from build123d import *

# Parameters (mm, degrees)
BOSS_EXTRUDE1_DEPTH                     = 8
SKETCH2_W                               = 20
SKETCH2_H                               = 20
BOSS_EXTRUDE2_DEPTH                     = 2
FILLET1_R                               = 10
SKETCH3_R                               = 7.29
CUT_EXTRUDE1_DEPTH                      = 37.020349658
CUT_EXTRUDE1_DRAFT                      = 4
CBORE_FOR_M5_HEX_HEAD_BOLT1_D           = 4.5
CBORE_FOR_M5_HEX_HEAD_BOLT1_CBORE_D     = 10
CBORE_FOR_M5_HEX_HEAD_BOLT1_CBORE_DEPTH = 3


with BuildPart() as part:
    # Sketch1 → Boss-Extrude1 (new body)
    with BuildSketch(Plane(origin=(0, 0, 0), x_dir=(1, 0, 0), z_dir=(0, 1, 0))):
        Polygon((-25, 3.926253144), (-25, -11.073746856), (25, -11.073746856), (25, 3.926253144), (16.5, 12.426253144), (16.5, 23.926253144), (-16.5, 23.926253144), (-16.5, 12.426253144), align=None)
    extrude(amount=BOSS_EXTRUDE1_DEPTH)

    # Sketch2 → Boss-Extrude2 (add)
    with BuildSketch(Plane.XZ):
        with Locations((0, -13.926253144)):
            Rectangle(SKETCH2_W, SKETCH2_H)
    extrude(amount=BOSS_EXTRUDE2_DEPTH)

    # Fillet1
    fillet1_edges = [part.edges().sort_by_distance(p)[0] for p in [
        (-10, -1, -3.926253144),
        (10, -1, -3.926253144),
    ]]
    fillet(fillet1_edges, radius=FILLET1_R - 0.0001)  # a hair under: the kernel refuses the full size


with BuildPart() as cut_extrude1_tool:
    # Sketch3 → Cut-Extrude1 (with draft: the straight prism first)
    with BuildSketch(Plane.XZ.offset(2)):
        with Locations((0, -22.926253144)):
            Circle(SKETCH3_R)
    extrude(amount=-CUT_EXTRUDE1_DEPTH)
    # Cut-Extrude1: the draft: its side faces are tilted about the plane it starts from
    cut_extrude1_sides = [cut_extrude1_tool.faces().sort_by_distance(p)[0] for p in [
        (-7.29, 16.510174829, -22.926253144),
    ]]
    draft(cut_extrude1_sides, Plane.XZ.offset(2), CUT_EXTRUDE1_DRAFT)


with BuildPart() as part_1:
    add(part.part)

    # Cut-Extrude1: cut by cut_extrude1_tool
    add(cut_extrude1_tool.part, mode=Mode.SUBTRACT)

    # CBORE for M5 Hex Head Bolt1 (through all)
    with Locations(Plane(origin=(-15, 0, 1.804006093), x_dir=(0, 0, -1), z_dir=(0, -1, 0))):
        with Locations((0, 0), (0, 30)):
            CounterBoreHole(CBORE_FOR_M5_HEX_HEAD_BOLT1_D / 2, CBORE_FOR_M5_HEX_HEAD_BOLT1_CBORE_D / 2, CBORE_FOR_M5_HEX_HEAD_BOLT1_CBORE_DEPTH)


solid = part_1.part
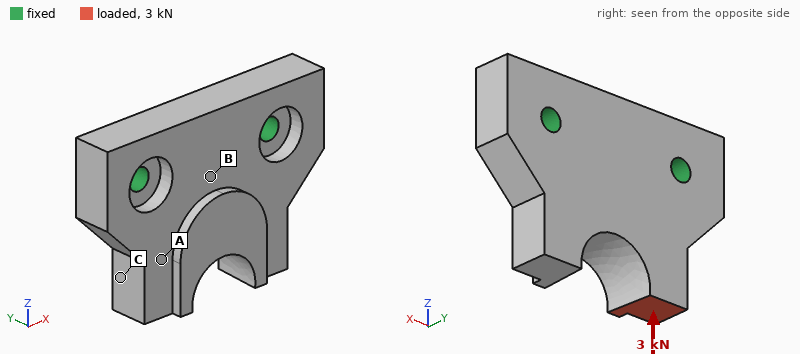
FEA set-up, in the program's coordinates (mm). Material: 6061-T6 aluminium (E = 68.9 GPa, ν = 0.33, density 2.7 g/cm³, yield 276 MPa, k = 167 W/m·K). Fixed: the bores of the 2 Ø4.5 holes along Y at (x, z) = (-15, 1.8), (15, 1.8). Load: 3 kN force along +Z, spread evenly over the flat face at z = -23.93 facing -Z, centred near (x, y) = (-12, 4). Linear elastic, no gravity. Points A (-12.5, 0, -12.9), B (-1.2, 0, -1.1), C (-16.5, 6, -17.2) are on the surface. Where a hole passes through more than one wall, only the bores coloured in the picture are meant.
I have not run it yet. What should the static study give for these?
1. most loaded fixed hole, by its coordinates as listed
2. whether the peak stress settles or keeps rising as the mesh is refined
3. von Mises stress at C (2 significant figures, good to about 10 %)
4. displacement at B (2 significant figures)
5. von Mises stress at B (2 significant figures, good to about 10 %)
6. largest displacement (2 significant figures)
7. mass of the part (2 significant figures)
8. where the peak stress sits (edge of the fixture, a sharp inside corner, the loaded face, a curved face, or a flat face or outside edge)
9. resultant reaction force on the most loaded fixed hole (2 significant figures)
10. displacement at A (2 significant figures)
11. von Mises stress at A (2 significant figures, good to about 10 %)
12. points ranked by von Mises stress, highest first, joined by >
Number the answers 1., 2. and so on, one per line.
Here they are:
1. (-15, 1.8)
2. keeps rising
3. 48 MPa
4. 6.3 µm
5. 10 MPa
6. 30 µm
7. 29 g
8. edge of the fixture
9. 2.6 kN
10. 16 µm
11. 29 MPa
12. C > A > B
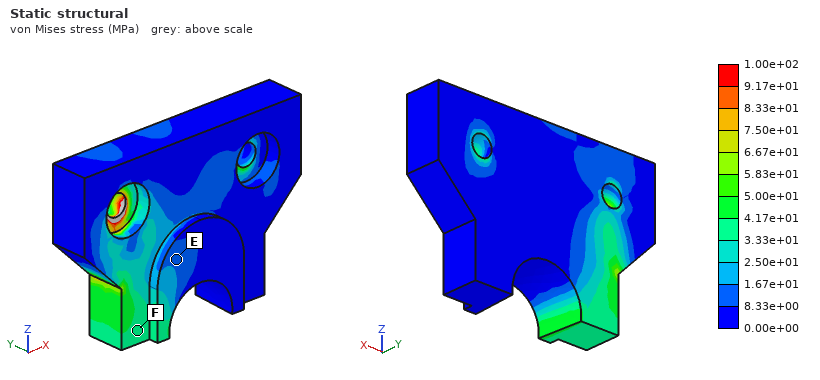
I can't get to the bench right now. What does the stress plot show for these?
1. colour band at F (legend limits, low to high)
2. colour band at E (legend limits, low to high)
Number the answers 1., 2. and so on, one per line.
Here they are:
1. 3.33e+01 to 4.17e+01 MPa
2. 8.33e+00 to 1.67e+01 MPa
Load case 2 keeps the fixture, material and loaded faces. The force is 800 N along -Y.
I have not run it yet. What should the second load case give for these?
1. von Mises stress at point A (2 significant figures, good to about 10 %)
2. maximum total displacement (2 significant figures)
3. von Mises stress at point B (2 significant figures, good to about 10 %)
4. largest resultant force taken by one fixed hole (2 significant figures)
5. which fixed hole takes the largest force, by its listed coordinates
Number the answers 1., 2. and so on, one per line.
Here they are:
1. 45 MPa
2. 0.11 mm
3. 32 MPa
4. 730 N
5. (-15, 1.8)
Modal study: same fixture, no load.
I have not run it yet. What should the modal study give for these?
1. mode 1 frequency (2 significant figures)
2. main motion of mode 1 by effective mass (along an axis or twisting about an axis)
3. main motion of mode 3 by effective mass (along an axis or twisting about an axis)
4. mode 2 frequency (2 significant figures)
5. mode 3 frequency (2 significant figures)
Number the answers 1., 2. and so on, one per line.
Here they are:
1. 7500 Hz
2. along Y
3. along Y
4. 16 kHz
5. 25 kHz
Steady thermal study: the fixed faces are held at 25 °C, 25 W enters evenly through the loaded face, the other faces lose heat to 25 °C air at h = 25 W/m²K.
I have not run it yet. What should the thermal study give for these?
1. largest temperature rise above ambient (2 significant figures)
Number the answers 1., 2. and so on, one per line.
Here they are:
1. 32 K
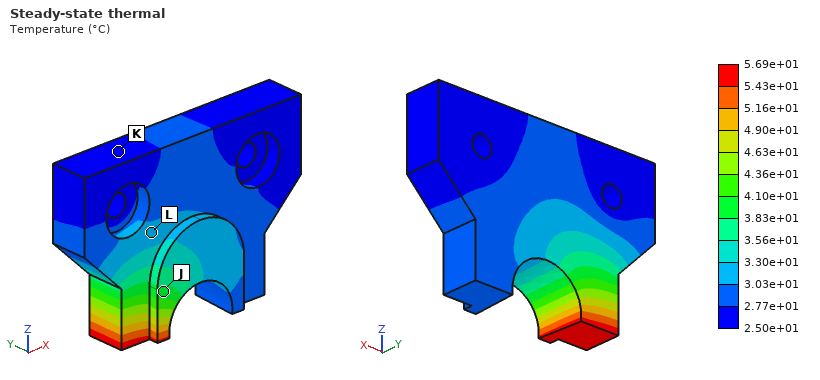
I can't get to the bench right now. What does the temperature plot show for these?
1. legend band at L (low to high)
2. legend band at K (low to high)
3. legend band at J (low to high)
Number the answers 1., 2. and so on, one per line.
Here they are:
1. 3.03e+01 to 3.30e+01 °C
2. 2.50e+01 to 2.77e+01 °C
3. 3.83e+01 to 4.10e+01 °C
